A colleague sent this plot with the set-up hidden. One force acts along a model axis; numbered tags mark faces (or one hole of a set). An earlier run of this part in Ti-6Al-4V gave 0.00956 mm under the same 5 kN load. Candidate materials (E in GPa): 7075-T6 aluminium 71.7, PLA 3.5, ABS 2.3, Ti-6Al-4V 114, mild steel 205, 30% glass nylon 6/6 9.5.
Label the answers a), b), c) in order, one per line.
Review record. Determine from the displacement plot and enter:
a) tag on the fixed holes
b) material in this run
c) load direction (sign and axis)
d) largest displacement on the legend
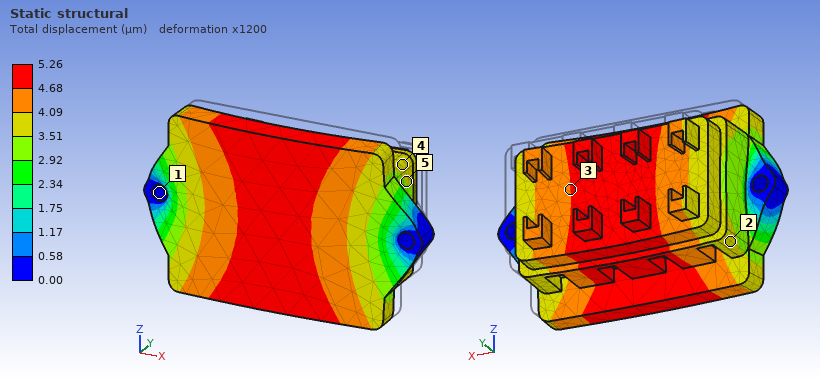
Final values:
a) 1
b) mild steel
c) -Y
d) 5.26 µm
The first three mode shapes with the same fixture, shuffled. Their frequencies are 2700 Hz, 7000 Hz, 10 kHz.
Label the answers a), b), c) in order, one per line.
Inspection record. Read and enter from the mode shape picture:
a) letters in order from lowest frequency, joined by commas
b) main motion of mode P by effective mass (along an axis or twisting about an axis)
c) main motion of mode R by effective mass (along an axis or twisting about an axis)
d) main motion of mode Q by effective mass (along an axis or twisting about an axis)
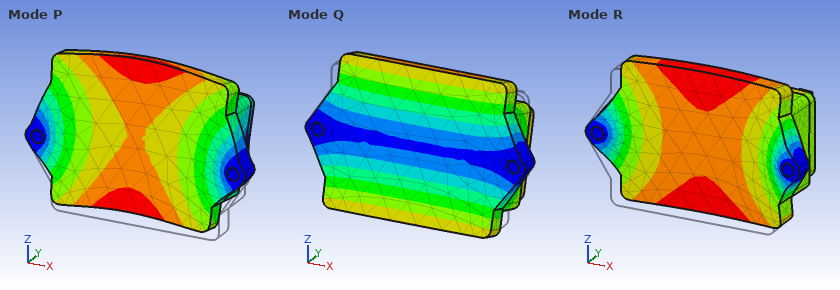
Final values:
a) Q, R, P
b) along Z
c) along Y
d) along Z
